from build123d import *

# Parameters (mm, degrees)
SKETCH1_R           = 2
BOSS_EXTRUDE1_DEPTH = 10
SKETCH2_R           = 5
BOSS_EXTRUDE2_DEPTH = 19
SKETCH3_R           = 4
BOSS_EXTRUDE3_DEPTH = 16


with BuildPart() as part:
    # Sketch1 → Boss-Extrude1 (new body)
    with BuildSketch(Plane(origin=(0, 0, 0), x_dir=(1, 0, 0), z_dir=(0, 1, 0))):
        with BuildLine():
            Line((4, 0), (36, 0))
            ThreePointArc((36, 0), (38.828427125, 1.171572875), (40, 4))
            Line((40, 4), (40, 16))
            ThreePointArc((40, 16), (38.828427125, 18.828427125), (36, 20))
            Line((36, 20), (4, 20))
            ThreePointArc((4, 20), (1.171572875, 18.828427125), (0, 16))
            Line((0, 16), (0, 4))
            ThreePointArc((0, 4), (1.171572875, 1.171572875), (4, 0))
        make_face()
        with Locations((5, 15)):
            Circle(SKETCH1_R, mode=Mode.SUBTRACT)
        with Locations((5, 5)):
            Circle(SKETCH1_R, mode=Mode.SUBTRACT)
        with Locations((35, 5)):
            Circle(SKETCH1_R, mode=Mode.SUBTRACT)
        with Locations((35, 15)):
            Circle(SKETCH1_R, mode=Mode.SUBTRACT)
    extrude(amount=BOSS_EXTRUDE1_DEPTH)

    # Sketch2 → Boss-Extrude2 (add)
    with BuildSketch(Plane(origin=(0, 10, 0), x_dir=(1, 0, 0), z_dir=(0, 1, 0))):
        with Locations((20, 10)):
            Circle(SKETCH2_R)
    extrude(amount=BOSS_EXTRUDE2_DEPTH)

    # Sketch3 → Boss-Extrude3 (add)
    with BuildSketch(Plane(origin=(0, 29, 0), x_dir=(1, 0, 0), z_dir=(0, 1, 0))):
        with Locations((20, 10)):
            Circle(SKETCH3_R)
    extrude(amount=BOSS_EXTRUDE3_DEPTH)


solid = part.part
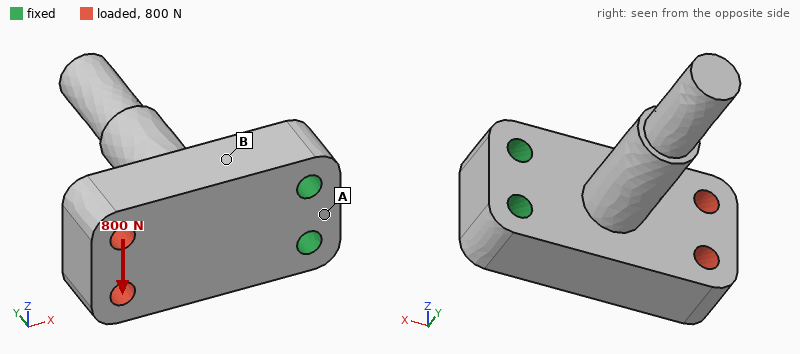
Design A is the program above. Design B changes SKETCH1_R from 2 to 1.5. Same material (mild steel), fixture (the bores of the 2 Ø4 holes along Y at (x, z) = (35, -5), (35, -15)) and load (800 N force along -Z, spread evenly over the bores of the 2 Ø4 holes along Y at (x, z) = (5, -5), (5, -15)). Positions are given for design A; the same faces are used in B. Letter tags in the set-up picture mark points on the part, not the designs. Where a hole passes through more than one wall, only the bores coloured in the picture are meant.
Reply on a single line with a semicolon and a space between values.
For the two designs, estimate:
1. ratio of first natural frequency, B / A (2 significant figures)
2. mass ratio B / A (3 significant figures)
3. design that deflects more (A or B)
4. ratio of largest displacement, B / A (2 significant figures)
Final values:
0.97; 1.02; B; 1.1
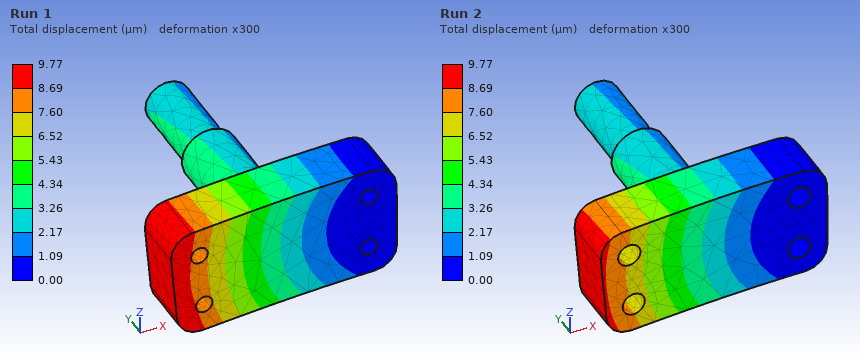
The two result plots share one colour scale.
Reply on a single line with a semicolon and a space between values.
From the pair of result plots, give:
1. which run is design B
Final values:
Run 1
